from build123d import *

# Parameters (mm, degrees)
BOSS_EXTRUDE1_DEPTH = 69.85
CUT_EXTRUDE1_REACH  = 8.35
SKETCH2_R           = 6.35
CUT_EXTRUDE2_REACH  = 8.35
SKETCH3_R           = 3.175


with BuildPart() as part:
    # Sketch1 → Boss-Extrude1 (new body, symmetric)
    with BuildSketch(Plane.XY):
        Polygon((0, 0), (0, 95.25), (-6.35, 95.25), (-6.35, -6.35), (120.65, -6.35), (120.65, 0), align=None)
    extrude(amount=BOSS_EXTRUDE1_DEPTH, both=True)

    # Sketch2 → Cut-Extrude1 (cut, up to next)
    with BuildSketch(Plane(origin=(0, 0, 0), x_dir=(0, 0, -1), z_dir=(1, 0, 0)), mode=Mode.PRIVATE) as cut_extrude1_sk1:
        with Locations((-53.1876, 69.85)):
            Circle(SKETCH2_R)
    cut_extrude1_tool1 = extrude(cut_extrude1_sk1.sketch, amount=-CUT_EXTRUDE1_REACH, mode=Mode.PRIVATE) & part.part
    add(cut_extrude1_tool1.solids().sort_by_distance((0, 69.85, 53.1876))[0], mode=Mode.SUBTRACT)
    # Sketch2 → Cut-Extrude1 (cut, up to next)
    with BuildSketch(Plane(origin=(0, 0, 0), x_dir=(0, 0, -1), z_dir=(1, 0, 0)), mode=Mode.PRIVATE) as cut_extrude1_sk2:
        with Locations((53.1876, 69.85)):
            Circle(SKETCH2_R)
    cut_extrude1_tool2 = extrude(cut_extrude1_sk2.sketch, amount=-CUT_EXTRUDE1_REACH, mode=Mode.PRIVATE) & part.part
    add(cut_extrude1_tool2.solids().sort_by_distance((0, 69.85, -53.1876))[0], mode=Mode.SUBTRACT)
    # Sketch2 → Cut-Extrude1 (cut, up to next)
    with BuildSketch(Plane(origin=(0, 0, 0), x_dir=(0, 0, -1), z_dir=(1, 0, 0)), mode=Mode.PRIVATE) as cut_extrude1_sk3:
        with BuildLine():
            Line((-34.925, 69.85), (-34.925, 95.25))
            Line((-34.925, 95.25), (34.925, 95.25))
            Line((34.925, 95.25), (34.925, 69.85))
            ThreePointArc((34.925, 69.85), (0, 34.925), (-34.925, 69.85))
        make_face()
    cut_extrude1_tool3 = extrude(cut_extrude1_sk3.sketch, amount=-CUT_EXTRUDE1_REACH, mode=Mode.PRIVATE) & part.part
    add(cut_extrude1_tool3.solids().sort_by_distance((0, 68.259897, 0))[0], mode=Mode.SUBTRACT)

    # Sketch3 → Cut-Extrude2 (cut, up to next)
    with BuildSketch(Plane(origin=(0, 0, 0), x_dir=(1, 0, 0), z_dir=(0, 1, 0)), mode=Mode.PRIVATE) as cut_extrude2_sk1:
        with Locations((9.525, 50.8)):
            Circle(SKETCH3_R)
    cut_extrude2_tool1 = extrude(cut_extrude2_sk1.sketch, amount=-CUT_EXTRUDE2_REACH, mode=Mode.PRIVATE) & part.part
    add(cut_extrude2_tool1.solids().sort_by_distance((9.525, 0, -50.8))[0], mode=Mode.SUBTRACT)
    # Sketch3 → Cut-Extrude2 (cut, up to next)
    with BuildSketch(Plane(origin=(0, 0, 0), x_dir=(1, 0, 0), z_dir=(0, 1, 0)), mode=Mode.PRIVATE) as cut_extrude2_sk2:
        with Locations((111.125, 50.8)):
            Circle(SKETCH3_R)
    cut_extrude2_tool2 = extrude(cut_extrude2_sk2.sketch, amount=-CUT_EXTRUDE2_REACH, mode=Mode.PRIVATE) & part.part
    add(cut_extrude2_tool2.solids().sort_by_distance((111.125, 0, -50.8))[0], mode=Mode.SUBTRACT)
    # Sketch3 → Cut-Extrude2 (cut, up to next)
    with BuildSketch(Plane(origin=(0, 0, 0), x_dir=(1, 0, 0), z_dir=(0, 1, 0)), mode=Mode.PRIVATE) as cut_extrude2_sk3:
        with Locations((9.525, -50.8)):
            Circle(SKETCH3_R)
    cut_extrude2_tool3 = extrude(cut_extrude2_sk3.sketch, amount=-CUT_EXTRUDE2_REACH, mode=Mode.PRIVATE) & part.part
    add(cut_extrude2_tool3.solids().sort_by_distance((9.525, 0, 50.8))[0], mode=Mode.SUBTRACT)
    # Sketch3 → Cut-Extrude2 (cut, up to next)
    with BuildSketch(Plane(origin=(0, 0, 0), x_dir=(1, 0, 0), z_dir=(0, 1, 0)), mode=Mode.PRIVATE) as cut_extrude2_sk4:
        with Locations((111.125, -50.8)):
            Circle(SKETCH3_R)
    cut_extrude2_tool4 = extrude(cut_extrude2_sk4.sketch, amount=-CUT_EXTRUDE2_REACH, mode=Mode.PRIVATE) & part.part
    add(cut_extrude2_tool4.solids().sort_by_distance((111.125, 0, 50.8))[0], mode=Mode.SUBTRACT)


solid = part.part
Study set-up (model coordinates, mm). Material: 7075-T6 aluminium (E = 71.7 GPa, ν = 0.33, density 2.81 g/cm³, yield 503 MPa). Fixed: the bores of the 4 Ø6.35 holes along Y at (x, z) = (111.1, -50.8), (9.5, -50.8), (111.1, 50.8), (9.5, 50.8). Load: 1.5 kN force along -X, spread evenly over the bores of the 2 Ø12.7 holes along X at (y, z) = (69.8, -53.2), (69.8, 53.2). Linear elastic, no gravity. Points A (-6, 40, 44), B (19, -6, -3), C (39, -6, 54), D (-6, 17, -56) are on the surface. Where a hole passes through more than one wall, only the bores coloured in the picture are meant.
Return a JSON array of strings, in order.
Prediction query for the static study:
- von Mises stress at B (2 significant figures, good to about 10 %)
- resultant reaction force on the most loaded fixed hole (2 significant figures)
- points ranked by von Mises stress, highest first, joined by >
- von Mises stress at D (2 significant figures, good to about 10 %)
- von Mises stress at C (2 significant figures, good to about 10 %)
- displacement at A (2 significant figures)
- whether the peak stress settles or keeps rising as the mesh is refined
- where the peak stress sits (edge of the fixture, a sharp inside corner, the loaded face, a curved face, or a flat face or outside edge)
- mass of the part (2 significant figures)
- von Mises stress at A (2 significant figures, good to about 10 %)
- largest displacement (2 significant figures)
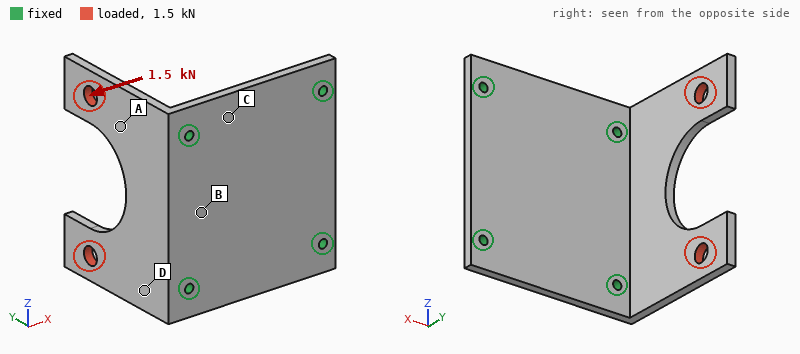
["43 MPa", "680 N", "D > A > B > C", "93 MPa", "16 MPa", "0.74 mm", "keeps rising", "edge of the fixture", "480 g", "72 MPa", "2.4 mm"]
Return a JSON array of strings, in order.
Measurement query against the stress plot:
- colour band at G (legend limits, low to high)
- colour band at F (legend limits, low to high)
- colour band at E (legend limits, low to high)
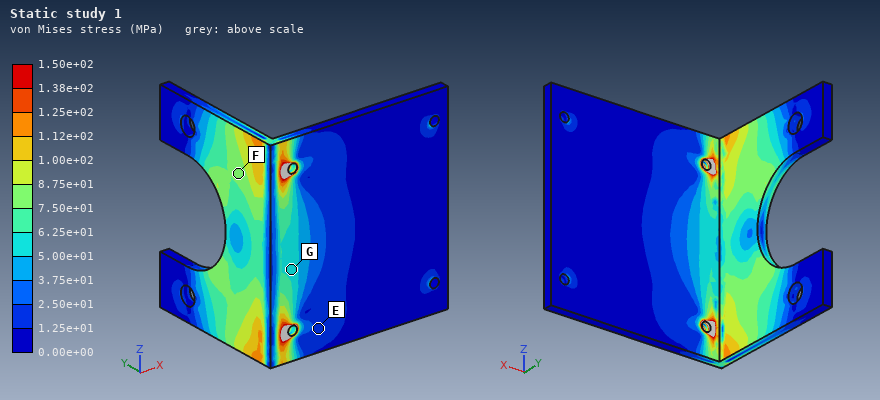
["5.00e+01 to 6.25e+01 MPa", "7.50e+01 to 8.75e+01 MPa", "1.25e+01 to 2.50e+01 MPa"]
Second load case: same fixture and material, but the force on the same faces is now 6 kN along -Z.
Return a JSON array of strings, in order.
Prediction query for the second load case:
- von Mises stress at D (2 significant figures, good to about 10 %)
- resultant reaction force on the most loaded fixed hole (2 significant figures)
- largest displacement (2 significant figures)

["25 MPa", "5.1 kN", "0.39 mm"]
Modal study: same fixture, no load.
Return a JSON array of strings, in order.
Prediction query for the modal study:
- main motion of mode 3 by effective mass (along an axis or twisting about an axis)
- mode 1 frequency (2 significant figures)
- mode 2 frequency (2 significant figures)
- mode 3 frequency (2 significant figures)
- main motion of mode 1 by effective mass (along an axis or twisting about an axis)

["along Y", "570 Hz", "680 Hz", "2200 Hz", "along X"]
